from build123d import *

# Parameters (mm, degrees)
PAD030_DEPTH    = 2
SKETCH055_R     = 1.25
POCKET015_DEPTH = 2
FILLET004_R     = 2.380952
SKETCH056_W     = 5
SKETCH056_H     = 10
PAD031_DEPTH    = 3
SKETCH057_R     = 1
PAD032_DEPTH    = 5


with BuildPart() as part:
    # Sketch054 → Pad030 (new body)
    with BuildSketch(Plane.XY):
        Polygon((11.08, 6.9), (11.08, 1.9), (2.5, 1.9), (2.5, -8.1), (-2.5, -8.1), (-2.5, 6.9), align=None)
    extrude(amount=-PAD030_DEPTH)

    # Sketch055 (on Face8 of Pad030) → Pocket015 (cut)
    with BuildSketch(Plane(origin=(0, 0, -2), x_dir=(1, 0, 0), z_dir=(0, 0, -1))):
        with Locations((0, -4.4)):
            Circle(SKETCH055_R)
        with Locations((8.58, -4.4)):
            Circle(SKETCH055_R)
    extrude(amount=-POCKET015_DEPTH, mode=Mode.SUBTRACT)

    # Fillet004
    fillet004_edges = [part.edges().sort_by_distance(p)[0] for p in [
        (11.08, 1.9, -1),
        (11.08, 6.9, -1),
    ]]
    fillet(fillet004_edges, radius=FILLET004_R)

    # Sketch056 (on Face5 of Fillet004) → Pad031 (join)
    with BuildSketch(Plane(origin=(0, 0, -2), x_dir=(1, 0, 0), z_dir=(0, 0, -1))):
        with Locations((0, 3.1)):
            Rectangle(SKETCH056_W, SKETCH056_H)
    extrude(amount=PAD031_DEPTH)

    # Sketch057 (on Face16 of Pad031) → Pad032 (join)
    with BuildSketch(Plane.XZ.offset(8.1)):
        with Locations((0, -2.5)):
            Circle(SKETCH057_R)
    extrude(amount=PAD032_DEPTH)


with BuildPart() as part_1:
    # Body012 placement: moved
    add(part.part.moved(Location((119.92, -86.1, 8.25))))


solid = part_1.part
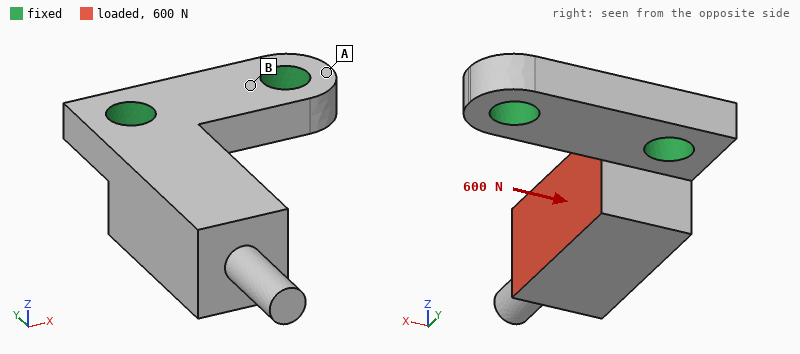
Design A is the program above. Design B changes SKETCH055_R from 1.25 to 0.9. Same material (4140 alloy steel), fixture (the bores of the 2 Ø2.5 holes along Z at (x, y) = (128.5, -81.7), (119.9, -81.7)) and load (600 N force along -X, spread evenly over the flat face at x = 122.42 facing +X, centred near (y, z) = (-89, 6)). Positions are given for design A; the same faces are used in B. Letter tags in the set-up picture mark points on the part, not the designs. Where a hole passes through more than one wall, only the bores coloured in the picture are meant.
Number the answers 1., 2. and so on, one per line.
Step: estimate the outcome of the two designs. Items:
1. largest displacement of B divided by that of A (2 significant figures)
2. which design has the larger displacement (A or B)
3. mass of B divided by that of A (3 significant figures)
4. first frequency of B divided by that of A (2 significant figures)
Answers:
1. 1.2
2. B
3. 1.03
4. 0.92
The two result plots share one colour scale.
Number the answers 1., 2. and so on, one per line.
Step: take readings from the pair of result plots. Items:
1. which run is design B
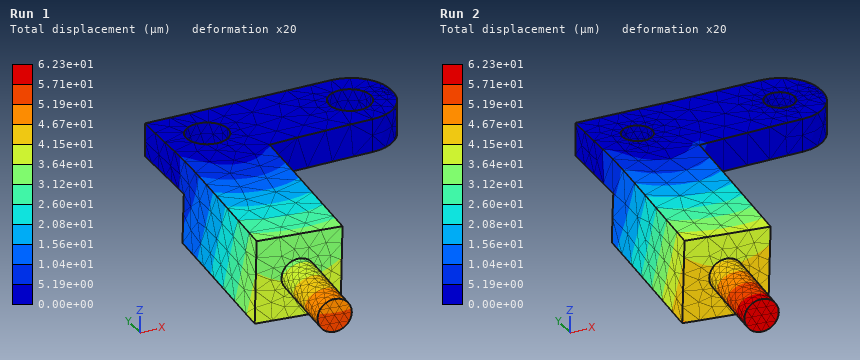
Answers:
1. Run 2
